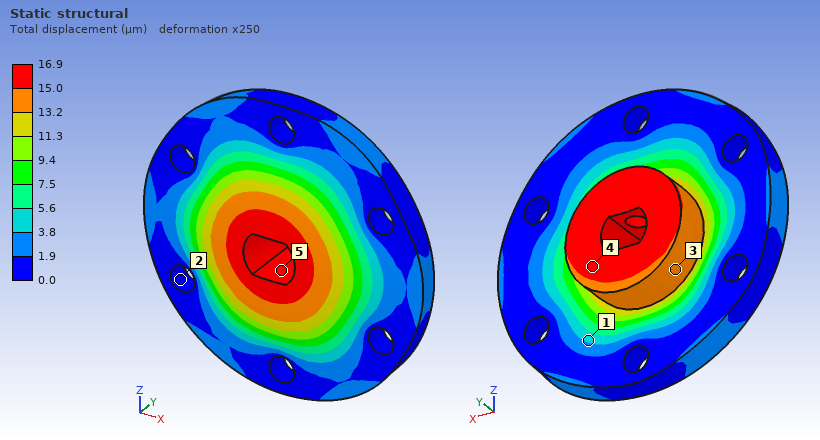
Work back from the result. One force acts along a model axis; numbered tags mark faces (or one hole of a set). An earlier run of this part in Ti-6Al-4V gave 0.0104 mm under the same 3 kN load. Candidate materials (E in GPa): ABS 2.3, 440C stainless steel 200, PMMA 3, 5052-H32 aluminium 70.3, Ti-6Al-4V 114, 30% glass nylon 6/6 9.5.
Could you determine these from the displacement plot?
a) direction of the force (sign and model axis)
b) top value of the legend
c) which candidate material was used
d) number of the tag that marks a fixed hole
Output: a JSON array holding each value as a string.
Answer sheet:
["-Y", "16.9 µm", "5052-H32 aluminium", "2"]
